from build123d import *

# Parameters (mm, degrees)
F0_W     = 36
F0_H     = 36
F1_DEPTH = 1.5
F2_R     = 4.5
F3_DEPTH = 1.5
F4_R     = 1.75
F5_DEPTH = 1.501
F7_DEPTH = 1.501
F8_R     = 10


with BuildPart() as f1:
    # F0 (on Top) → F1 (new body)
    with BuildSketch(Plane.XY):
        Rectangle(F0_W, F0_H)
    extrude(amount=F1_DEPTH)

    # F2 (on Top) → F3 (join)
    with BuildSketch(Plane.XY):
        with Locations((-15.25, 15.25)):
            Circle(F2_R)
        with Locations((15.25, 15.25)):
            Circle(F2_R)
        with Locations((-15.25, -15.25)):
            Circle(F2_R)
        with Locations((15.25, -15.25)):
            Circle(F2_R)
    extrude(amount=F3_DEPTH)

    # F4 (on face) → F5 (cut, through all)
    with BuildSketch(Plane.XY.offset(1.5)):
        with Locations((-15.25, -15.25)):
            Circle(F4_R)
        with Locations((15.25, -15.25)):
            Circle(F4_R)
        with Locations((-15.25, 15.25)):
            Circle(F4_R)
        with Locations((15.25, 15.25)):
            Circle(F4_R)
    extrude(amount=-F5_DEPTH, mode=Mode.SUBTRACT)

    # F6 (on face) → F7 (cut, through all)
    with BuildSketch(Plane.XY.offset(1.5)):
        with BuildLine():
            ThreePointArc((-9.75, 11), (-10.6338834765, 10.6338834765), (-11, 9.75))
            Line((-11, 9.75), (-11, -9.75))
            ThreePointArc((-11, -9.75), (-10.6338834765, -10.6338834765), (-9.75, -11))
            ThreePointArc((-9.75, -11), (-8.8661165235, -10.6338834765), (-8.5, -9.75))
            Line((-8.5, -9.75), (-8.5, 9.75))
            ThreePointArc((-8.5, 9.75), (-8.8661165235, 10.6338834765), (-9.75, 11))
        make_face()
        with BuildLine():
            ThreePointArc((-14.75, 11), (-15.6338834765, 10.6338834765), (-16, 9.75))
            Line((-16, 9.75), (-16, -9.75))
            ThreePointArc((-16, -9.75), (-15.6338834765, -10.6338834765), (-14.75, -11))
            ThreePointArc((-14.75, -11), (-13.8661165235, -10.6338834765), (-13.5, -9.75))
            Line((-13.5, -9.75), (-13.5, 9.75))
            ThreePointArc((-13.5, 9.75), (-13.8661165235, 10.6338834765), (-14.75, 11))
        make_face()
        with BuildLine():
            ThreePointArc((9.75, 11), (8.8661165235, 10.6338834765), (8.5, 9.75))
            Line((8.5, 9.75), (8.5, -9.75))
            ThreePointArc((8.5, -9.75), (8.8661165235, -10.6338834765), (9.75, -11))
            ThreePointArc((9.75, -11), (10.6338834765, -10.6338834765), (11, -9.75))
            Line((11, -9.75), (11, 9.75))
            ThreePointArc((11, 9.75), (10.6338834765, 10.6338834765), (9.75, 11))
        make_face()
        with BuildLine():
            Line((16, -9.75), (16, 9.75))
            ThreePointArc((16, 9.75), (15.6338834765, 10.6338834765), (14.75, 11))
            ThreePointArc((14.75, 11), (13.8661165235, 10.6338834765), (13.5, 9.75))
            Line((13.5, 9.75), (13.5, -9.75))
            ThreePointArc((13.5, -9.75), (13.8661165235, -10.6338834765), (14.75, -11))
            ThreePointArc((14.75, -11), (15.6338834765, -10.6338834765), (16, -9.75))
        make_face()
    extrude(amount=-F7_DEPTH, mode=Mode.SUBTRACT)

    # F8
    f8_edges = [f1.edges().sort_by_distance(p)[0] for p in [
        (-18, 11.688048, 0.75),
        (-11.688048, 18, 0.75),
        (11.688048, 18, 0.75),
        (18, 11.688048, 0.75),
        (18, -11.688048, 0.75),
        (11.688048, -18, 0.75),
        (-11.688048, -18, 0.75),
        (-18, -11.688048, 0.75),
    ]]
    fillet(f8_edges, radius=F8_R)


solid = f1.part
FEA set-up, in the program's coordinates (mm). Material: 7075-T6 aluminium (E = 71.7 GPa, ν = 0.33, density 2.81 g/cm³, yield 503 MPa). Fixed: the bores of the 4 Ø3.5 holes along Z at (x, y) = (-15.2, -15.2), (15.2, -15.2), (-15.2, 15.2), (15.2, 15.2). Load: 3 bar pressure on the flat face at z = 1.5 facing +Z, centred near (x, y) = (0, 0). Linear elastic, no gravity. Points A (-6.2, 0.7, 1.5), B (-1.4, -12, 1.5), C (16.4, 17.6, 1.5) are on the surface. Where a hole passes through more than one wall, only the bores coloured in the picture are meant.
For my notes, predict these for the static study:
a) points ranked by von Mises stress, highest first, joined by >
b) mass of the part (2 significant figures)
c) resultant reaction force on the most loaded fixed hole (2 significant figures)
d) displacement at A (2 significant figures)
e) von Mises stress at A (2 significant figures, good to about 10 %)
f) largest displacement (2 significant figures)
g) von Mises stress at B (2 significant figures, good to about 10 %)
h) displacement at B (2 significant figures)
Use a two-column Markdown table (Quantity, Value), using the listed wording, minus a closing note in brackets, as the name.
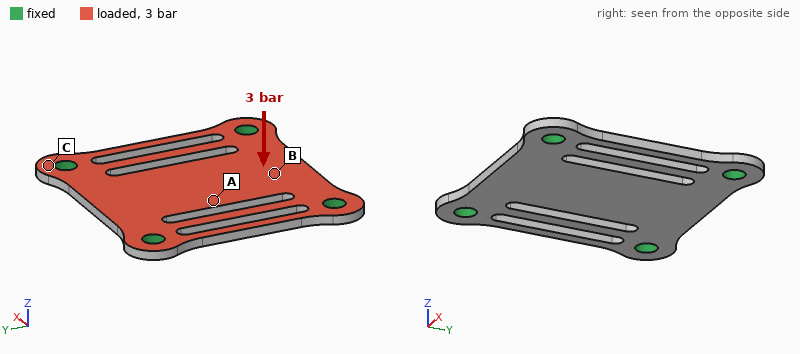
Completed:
| Quantity | Value |
|---|---|
| points ranked by von Mises stress, highest first, joined by > | A > B > C |
| mass of the part | 4.7 g |
| resultant reaction force on the most loaded fixed hole | 84 N |
| displacement at A | 78 µm |
| von Mises stress at A | 41 MPa |
| largest displacement | 81 µm |
| von Mises stress at B | 31 MPa |
| displacement at B | 48 µm |
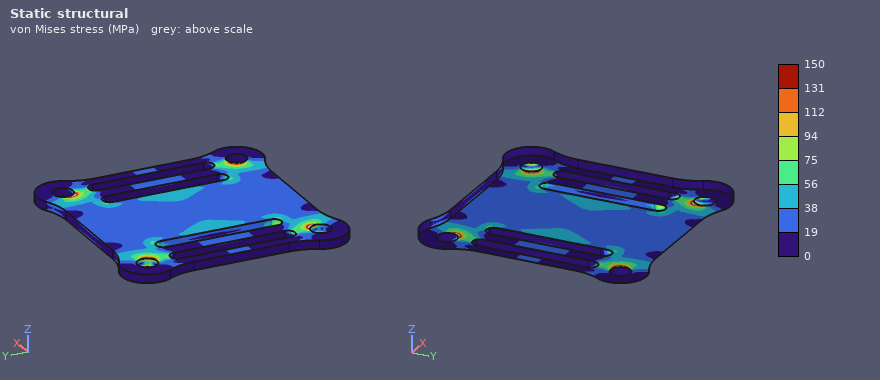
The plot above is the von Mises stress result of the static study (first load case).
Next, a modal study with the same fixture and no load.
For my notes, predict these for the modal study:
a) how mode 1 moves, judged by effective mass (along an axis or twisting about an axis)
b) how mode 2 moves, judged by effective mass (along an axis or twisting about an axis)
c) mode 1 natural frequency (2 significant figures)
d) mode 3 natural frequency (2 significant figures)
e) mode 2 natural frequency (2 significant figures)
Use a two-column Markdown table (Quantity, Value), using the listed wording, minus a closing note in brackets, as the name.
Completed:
| Quantity | Value |
|---|---|
| how mode 1 moves, judged by effective mass | along Z |
| how mode 2 moves, judged by effective mass | twisting about X |
| mode 1 natural frequency | 5500 Hz |
| mode 3 natural frequency | 11 kHz |
| mode 2 natural frequency | 10 kHz |
